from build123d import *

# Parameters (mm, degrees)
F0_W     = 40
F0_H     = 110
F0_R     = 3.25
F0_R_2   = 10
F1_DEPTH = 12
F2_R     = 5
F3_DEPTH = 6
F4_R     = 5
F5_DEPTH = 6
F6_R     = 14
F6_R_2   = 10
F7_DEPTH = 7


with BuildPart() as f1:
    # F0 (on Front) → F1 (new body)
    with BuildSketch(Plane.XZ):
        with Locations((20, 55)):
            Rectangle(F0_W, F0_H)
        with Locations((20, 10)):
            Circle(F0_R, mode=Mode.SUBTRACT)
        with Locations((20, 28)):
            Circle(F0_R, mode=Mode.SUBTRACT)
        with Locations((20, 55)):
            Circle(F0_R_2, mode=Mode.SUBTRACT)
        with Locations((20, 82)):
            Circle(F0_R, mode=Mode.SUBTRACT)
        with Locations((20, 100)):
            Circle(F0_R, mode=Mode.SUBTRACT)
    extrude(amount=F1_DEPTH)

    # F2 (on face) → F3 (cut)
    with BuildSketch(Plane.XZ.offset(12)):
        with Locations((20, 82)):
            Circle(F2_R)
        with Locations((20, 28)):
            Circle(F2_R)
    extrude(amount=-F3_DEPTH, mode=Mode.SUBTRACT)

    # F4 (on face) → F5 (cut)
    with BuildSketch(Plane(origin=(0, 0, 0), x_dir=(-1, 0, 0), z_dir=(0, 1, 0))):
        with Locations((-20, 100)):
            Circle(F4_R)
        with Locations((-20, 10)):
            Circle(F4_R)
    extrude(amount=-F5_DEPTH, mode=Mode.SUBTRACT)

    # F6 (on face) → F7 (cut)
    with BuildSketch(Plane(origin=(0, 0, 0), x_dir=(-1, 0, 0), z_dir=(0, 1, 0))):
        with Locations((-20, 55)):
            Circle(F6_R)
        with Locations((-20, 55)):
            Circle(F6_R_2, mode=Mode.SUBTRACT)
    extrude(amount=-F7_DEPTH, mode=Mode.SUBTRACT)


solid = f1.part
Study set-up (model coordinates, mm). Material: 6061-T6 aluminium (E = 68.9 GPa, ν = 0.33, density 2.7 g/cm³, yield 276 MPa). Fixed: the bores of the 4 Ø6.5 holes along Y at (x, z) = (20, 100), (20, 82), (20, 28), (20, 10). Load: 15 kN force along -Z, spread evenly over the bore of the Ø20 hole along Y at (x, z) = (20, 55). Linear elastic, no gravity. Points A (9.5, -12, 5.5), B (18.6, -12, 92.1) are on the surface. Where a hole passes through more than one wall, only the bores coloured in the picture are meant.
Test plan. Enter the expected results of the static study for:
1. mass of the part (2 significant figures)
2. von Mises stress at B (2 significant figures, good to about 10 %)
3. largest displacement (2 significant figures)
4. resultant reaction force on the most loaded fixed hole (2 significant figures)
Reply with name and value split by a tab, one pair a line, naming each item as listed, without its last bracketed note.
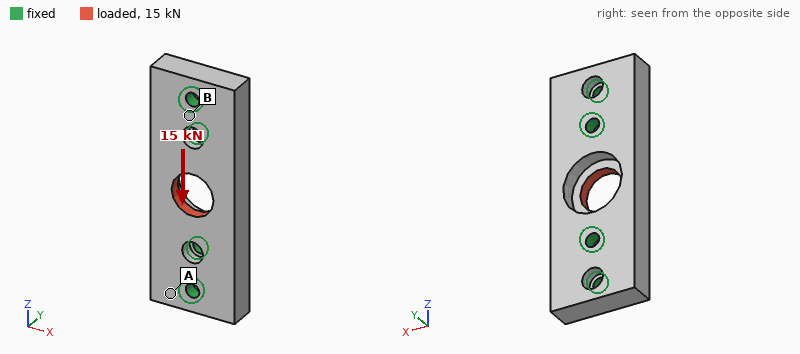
mass of the part	120 g
von Mises stress at B	18 MPa
largest displacement	20 µm
resultant reaction force on the most loaded fixed hole	5.1 kN
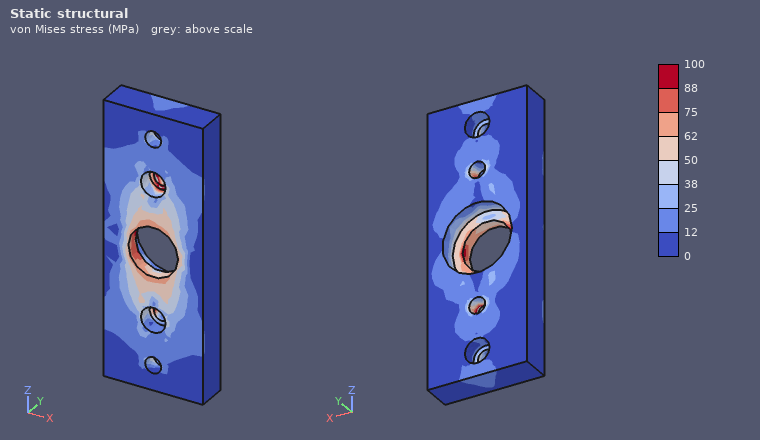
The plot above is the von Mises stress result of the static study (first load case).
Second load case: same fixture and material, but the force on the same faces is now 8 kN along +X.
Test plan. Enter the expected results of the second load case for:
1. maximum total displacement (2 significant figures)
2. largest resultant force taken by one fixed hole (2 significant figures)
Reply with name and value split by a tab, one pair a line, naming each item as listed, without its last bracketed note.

maximum total displacement	43 µm
largest resultant force taken by one fixed hole	3.6 kN
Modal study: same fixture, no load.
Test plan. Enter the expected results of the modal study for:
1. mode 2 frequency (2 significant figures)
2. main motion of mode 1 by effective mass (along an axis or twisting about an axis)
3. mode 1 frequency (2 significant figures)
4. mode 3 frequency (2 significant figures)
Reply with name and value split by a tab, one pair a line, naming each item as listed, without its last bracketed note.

mode 2 frequency	13 kHz
main motion of mode 1 by effective mass	twisting about Z
mode 1 frequency	8900 Hz
mode 3 frequency	13 kHz
